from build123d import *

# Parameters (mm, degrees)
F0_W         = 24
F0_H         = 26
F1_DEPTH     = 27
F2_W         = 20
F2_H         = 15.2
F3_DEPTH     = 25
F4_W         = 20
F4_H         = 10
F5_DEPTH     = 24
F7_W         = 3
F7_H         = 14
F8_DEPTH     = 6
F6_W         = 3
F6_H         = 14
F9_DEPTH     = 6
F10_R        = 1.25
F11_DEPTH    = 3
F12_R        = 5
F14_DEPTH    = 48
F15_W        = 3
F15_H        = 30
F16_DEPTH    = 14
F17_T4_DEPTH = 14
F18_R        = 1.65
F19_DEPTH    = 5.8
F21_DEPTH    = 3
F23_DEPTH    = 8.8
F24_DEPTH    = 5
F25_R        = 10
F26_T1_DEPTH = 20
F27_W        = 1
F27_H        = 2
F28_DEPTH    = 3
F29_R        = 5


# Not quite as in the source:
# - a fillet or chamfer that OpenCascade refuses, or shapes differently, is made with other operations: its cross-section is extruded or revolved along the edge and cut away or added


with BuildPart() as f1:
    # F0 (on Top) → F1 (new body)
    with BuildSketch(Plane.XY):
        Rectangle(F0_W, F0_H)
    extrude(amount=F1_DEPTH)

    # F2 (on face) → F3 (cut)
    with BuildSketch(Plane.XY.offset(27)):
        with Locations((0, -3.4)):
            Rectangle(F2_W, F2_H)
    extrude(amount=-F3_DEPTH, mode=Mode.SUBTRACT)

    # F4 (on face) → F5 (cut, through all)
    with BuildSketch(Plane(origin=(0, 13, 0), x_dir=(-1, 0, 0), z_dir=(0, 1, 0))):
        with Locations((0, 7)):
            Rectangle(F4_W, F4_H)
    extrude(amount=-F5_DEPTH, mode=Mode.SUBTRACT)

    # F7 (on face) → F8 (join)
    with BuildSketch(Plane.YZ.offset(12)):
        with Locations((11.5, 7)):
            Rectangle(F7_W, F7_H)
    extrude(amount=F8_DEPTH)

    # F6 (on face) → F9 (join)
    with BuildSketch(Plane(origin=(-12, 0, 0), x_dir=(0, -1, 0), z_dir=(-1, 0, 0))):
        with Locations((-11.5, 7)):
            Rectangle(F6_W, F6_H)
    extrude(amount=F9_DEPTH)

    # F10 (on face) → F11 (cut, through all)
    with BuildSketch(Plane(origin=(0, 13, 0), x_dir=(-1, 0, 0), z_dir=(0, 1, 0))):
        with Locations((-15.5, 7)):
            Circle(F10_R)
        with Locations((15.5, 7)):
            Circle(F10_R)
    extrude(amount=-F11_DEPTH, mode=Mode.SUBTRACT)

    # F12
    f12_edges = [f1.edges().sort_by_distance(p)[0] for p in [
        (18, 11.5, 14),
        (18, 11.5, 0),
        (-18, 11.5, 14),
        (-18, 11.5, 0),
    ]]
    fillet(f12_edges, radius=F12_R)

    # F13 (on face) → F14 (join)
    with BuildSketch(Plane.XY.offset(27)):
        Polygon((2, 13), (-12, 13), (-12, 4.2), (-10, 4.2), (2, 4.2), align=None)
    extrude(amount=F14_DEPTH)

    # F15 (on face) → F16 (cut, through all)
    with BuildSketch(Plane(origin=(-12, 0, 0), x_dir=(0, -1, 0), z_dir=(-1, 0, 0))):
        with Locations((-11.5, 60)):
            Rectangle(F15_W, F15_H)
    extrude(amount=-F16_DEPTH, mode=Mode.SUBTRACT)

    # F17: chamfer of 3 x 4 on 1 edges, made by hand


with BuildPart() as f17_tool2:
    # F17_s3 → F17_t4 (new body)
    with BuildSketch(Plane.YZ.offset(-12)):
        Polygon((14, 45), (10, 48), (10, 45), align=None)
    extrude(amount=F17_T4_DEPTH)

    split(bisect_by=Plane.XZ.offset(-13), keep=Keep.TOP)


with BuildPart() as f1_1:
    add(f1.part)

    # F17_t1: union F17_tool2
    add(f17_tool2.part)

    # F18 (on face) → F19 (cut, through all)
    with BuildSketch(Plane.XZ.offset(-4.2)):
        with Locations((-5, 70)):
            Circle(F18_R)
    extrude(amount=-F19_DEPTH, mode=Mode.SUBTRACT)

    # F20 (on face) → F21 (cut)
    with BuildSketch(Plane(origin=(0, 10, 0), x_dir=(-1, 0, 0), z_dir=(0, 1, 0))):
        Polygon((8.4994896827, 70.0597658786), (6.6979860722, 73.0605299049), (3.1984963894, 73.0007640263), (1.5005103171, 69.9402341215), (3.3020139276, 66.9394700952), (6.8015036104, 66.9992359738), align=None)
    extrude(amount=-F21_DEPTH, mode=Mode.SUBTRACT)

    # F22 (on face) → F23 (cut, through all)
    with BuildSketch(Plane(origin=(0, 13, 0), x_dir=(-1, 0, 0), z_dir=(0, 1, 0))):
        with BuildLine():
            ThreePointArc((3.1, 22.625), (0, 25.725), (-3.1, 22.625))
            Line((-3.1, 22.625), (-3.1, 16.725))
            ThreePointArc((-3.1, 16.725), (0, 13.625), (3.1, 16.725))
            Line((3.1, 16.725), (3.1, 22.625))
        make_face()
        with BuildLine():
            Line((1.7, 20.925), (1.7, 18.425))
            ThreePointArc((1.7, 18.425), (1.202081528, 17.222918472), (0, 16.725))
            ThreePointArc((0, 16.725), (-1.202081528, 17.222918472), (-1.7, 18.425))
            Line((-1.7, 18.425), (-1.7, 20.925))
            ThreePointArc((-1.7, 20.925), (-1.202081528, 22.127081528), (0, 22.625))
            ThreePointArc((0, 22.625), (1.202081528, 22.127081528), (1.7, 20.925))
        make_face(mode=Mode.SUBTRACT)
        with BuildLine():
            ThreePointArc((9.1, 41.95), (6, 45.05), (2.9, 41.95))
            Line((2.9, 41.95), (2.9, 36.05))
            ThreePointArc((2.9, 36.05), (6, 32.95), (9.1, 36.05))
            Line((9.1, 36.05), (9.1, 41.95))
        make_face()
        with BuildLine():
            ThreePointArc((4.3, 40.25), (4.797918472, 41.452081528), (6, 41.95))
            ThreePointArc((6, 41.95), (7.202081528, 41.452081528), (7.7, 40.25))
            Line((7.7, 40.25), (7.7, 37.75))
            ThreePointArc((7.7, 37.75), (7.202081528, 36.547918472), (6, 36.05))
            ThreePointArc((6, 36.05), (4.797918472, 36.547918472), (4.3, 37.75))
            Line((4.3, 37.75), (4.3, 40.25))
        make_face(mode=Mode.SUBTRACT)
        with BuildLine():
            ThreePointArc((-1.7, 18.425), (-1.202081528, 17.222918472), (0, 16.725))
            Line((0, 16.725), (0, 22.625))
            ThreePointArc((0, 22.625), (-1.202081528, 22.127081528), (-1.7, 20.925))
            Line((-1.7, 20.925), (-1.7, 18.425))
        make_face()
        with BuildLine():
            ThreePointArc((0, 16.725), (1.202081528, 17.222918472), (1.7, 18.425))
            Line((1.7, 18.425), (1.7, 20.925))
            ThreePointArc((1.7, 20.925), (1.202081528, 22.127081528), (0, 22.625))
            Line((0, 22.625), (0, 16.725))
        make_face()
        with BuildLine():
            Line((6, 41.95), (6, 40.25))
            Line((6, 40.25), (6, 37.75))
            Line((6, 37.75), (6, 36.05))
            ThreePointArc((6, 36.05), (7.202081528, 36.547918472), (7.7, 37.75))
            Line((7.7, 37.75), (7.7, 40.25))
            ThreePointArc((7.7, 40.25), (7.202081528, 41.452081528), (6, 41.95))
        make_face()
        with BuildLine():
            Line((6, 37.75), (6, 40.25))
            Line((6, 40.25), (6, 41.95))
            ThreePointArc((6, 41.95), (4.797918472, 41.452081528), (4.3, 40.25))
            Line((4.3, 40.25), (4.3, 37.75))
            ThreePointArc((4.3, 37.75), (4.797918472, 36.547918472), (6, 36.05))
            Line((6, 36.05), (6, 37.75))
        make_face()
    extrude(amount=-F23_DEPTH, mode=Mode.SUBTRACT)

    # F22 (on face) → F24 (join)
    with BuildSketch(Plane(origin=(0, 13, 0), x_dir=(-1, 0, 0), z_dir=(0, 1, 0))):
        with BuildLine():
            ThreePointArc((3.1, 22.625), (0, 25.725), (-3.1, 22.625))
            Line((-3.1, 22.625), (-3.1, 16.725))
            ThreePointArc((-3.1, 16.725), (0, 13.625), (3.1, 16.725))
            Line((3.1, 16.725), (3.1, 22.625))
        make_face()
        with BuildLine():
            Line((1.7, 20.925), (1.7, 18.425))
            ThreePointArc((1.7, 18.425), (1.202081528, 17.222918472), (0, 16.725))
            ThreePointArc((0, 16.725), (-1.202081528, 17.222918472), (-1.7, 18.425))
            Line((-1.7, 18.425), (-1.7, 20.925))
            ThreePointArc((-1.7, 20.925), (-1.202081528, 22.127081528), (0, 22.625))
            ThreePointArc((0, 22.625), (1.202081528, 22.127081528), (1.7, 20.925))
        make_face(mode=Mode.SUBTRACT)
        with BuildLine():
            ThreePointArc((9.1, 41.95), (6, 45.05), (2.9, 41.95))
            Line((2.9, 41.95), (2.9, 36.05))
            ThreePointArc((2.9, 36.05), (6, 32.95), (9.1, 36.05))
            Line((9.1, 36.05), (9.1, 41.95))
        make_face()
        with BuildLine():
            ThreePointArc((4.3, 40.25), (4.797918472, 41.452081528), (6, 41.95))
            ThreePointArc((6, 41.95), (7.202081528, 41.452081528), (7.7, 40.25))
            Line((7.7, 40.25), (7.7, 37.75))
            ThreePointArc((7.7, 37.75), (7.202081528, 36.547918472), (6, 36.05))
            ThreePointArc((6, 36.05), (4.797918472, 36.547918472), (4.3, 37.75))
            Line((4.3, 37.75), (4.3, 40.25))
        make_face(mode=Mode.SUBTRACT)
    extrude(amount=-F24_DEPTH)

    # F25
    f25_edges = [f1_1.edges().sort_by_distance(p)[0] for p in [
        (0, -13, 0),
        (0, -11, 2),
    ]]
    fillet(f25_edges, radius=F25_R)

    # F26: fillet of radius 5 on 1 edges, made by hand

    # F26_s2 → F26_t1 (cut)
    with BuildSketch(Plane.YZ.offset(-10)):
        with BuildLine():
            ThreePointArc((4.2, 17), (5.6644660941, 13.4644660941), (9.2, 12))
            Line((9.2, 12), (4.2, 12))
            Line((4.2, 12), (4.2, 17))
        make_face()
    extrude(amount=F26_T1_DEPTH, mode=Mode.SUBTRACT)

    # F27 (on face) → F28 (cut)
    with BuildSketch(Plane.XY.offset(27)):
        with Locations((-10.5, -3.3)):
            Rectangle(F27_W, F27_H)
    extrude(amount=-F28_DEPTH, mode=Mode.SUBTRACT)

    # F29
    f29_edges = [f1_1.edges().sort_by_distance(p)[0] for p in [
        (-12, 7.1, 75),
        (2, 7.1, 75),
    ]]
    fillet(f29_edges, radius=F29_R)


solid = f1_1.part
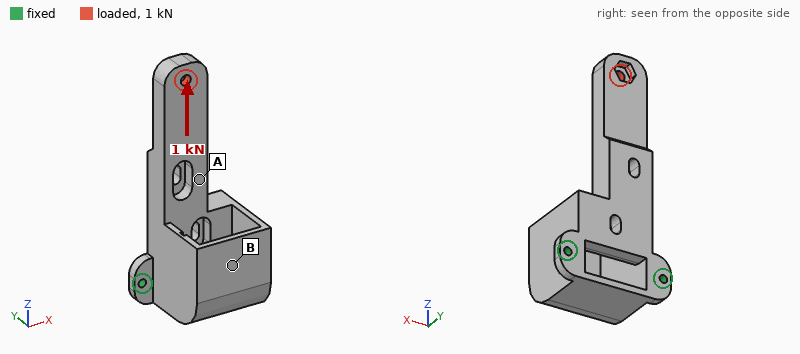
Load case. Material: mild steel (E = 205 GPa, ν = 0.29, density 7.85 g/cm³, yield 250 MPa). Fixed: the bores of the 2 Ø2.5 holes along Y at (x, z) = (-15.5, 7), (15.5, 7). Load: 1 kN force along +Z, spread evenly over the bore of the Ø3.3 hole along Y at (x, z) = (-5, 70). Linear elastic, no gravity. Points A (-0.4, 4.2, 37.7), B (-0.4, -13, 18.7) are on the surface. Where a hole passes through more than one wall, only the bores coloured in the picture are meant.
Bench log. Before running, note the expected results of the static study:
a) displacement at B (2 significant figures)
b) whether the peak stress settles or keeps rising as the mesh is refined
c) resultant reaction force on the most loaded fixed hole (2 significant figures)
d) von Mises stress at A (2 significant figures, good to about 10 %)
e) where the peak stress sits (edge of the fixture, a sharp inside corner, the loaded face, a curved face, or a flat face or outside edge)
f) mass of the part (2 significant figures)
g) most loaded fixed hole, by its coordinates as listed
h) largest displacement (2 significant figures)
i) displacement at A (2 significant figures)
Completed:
0.045 mm
keeps rising
700 N
39 MPa
edge of the fixture
91 g
(-15.5, 7)
0.16 mm
0.057 mm
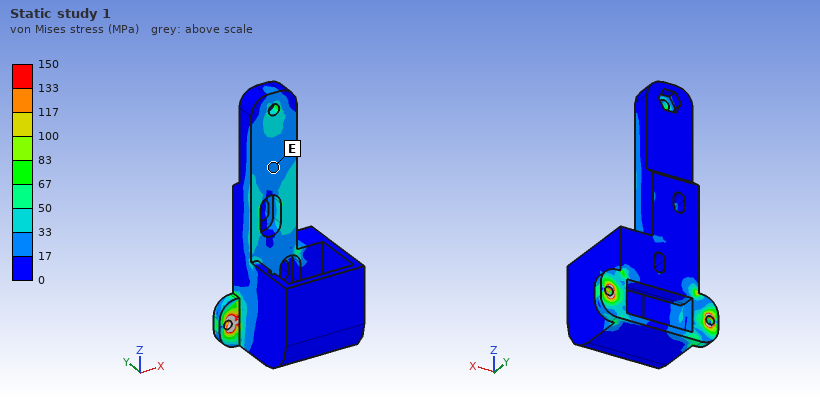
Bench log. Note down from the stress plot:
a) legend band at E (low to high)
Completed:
17 to 33 MPa
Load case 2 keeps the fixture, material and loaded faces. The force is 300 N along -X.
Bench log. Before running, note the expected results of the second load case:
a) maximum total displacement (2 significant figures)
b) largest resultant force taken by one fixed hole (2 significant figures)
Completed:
63 µm
720 N
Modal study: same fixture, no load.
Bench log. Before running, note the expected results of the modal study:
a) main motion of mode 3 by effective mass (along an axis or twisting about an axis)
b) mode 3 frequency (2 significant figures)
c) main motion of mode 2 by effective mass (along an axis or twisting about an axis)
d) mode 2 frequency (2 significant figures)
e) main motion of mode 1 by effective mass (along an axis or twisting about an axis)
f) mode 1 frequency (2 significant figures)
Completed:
along Z
4800 Hz
along X
3500 Hz
along Y
1000 Hz
